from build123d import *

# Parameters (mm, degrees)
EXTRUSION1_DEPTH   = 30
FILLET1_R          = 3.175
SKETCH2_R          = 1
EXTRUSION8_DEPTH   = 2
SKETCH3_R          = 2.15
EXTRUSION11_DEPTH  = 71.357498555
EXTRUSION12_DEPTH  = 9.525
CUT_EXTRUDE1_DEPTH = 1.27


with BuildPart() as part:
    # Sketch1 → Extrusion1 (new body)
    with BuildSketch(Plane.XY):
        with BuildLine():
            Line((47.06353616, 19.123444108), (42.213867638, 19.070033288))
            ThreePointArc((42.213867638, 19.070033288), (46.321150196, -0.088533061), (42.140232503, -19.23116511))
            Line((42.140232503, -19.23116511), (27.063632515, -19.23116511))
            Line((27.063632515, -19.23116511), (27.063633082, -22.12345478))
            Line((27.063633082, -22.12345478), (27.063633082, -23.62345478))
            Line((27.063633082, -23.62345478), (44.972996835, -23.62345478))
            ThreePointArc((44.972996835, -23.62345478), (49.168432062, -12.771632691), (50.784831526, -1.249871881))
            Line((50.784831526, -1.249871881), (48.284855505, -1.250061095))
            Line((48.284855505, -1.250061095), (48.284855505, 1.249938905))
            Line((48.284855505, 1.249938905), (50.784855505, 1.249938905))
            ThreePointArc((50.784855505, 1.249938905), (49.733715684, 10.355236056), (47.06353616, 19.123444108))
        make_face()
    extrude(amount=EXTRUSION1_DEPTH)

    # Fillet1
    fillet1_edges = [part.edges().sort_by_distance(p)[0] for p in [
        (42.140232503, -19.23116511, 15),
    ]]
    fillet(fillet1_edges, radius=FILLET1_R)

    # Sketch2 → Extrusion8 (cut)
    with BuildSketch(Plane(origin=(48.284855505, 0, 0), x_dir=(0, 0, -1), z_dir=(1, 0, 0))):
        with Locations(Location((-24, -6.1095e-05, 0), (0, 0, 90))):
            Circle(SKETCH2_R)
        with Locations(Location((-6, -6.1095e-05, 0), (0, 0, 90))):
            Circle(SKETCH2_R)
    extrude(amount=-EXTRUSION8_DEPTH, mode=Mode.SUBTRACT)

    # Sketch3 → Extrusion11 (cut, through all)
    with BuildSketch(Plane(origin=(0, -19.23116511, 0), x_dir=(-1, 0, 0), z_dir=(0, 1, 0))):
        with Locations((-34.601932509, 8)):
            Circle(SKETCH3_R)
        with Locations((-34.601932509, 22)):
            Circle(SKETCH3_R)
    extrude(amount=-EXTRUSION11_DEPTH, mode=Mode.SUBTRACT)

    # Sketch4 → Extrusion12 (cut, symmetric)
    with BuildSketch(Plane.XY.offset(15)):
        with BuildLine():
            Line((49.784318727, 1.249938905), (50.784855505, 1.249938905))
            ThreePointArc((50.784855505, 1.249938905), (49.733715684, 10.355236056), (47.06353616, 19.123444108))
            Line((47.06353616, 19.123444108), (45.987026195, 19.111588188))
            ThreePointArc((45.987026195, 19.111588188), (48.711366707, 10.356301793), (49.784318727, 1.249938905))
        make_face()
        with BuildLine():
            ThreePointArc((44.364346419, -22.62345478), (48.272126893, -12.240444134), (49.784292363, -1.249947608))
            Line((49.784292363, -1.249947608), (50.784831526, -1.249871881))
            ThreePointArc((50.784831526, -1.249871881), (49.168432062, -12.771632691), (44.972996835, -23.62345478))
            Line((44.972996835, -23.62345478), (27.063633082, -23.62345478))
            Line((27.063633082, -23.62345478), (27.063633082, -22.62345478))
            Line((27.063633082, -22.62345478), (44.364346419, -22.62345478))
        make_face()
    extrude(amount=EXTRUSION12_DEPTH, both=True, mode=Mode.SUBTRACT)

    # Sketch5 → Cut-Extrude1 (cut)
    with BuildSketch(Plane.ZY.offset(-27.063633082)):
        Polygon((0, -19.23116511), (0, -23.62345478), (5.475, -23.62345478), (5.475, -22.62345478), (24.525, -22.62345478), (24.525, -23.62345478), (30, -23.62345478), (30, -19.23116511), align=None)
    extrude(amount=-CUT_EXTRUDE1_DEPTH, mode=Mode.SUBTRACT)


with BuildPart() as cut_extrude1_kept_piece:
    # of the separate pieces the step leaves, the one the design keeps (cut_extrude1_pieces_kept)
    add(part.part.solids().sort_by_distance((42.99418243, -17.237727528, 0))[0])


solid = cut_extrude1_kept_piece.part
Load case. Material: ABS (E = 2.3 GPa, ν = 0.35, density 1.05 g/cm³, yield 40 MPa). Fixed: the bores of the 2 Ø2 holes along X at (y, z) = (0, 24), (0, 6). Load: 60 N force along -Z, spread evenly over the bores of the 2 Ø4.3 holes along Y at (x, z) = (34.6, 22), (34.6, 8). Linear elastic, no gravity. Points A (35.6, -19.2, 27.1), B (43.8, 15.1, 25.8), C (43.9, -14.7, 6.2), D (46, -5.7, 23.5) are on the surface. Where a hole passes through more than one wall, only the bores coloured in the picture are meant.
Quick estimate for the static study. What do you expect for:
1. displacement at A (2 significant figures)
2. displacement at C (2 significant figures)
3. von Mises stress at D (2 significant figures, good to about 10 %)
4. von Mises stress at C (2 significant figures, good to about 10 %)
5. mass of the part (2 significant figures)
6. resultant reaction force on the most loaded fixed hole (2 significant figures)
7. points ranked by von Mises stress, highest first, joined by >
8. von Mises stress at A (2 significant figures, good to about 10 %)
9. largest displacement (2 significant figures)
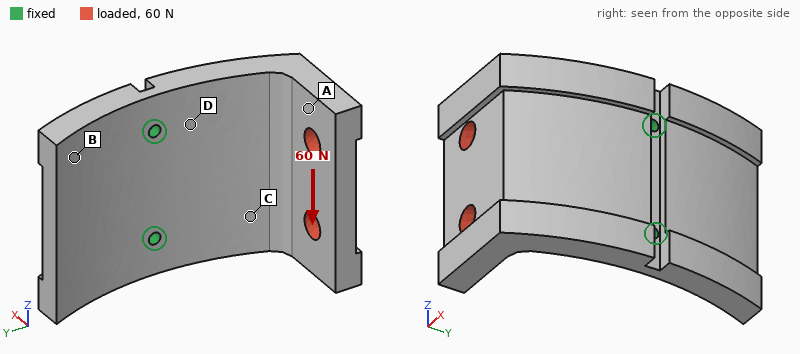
0.43 mm
0.19 mm
8.7 MPa
6.7 MPa
6.6 g
83 N
D > C > A > B
2.9 MPa
0.63 mm
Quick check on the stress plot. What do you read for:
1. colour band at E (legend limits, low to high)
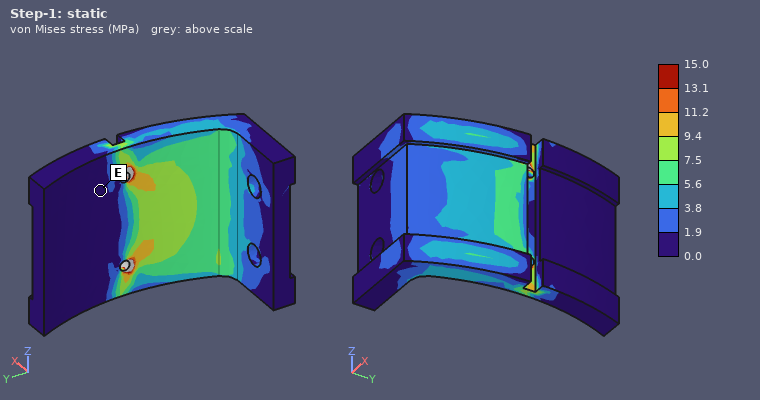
0.0 to 1.9 MPa
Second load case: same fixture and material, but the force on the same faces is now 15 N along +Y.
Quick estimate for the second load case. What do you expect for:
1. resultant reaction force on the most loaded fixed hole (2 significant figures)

8.4 N
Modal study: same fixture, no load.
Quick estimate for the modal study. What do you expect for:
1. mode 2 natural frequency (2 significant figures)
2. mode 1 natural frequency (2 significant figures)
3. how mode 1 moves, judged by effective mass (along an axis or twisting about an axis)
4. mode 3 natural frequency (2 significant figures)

1200 Hz
500 Hz
along X
1200 Hz
